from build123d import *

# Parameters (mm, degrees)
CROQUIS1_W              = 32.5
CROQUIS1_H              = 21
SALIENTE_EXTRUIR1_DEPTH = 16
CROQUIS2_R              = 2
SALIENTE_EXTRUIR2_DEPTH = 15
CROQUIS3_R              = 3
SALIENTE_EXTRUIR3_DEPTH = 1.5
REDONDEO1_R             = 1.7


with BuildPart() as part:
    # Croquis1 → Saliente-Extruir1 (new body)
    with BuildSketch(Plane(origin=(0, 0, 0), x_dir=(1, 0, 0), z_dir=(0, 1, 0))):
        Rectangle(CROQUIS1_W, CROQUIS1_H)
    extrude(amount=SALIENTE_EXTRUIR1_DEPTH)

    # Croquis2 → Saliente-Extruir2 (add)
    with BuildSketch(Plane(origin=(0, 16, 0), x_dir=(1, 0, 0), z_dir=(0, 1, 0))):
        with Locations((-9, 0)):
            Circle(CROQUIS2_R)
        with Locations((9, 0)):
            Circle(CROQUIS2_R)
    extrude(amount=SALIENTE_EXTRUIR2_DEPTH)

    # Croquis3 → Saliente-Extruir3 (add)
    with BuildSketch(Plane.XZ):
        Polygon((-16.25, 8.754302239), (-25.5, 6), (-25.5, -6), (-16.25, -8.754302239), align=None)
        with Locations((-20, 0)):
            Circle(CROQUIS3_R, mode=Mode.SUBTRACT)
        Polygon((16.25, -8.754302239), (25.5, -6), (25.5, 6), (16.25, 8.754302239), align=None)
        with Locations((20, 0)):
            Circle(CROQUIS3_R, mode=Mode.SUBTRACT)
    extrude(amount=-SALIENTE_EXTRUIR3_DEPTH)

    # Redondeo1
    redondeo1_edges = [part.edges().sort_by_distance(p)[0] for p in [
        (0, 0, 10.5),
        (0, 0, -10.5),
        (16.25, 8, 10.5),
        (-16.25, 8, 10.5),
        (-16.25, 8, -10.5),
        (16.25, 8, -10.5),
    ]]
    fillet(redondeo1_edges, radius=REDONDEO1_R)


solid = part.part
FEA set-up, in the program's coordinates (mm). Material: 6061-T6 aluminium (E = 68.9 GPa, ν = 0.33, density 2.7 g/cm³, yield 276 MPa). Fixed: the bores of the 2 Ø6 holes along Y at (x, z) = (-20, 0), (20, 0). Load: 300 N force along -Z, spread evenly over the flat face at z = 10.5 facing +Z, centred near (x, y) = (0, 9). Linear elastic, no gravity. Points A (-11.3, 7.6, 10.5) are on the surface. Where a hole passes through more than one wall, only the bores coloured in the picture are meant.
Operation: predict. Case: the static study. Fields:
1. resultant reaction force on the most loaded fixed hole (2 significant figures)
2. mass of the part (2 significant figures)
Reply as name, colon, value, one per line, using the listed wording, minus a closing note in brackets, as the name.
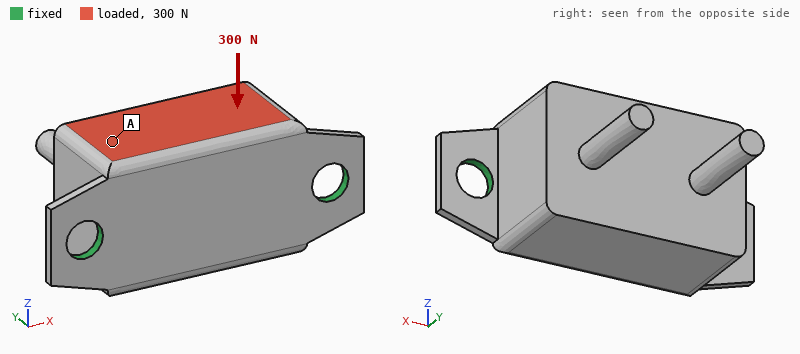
resultant reaction force on the most loaded fixed hole: 150 N
mass of the part: 31 g
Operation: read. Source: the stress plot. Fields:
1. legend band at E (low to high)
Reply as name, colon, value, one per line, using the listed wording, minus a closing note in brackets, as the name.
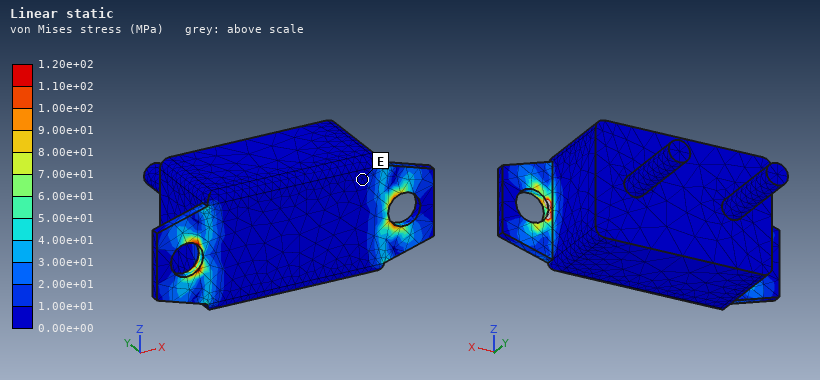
legend band at E: 0.00e+00 to 1.00e+01 MPa
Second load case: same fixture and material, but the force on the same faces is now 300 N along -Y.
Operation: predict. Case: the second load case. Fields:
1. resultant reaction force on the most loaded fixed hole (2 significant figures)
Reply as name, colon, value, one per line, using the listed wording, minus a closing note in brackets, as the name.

resultant reaction force on the most loaded fixed hole: 180 N
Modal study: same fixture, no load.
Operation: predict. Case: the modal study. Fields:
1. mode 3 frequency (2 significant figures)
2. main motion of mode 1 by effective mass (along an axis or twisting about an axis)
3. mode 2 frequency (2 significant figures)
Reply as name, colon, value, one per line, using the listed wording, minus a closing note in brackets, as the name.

mode 3 frequency: 11 kHz
main motion of mode 1 by effective mass: along Z
mode 2 frequency: 10 kHz
